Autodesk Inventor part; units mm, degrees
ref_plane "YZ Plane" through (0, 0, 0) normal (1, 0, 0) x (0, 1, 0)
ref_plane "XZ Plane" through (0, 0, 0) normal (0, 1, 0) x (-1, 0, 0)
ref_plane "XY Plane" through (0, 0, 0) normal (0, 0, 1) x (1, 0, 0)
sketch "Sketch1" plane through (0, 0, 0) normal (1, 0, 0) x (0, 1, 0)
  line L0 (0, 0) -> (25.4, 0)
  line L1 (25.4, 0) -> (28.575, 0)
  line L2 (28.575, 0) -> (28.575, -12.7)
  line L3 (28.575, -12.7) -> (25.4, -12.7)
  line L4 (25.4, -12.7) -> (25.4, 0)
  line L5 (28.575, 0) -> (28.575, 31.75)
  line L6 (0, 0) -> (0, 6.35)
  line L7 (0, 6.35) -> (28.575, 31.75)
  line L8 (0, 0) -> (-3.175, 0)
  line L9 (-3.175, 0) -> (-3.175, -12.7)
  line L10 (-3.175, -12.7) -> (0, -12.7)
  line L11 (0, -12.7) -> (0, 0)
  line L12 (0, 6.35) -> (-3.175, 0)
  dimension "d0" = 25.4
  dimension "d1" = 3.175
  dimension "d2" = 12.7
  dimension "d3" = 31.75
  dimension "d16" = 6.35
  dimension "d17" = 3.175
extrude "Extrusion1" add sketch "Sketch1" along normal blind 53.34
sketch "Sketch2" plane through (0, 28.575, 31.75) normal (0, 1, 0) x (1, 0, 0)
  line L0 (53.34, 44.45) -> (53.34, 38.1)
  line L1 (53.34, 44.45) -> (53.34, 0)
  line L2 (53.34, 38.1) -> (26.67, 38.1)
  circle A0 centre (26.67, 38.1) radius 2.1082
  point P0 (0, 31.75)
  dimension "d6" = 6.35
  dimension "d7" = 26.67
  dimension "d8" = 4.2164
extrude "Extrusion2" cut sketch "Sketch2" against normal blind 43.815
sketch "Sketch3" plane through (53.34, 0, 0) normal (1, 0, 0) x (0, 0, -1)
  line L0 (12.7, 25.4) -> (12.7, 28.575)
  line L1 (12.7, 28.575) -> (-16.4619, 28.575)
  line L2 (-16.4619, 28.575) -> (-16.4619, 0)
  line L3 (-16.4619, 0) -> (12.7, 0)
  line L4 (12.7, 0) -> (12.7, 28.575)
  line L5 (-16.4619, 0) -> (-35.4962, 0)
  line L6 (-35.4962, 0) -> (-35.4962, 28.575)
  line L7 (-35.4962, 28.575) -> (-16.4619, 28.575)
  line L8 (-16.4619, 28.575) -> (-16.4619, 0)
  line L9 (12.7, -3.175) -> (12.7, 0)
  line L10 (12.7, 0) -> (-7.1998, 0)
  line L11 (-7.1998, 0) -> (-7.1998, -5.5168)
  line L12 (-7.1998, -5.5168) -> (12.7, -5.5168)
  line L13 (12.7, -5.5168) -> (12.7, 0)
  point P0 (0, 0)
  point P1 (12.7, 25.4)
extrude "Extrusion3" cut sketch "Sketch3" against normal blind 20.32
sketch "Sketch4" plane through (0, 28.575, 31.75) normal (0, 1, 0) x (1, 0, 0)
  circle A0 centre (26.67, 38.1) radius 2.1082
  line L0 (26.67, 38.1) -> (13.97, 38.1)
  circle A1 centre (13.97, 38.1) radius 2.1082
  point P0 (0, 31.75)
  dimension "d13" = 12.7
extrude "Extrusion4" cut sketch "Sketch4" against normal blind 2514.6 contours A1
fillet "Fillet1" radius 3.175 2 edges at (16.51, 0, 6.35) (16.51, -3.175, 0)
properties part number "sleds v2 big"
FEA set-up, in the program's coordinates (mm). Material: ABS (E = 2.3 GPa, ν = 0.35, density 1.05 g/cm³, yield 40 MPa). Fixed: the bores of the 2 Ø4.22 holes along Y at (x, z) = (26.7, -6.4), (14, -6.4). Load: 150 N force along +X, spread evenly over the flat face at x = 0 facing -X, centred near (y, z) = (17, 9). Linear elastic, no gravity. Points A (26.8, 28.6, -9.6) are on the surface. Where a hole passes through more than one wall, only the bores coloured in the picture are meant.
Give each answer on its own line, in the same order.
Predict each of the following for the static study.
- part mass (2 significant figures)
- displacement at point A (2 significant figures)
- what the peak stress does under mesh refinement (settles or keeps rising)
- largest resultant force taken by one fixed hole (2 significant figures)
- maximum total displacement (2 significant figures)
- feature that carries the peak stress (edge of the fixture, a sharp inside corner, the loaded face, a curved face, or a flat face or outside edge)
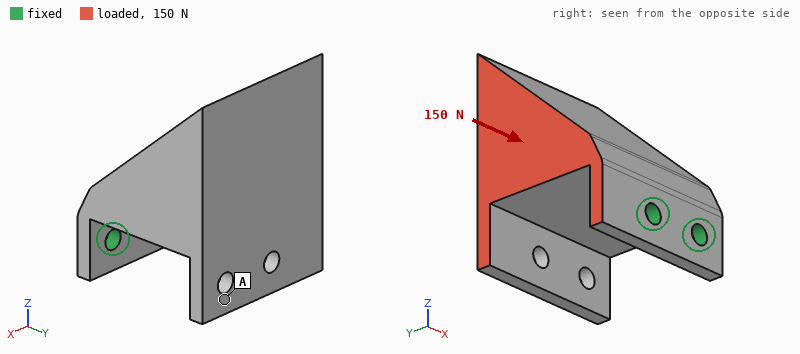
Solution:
22 g
0.53 mm
keeps rising
230 N
0.65 mm
edge of the fixture
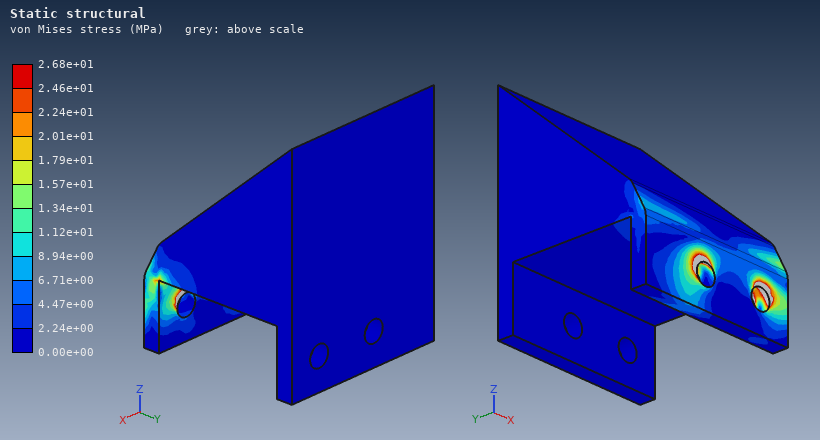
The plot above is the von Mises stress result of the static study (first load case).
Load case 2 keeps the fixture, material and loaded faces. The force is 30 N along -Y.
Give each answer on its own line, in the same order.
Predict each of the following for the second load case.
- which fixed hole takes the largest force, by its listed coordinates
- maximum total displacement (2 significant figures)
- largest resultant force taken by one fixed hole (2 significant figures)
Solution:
(14, -6.4)
0.72 mm
50 N
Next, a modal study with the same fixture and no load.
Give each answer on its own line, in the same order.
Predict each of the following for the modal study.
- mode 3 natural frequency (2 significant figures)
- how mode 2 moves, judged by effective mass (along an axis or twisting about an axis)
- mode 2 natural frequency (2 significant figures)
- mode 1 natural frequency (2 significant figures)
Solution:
1600 Hz
along X
620 Hz
210 Hz
